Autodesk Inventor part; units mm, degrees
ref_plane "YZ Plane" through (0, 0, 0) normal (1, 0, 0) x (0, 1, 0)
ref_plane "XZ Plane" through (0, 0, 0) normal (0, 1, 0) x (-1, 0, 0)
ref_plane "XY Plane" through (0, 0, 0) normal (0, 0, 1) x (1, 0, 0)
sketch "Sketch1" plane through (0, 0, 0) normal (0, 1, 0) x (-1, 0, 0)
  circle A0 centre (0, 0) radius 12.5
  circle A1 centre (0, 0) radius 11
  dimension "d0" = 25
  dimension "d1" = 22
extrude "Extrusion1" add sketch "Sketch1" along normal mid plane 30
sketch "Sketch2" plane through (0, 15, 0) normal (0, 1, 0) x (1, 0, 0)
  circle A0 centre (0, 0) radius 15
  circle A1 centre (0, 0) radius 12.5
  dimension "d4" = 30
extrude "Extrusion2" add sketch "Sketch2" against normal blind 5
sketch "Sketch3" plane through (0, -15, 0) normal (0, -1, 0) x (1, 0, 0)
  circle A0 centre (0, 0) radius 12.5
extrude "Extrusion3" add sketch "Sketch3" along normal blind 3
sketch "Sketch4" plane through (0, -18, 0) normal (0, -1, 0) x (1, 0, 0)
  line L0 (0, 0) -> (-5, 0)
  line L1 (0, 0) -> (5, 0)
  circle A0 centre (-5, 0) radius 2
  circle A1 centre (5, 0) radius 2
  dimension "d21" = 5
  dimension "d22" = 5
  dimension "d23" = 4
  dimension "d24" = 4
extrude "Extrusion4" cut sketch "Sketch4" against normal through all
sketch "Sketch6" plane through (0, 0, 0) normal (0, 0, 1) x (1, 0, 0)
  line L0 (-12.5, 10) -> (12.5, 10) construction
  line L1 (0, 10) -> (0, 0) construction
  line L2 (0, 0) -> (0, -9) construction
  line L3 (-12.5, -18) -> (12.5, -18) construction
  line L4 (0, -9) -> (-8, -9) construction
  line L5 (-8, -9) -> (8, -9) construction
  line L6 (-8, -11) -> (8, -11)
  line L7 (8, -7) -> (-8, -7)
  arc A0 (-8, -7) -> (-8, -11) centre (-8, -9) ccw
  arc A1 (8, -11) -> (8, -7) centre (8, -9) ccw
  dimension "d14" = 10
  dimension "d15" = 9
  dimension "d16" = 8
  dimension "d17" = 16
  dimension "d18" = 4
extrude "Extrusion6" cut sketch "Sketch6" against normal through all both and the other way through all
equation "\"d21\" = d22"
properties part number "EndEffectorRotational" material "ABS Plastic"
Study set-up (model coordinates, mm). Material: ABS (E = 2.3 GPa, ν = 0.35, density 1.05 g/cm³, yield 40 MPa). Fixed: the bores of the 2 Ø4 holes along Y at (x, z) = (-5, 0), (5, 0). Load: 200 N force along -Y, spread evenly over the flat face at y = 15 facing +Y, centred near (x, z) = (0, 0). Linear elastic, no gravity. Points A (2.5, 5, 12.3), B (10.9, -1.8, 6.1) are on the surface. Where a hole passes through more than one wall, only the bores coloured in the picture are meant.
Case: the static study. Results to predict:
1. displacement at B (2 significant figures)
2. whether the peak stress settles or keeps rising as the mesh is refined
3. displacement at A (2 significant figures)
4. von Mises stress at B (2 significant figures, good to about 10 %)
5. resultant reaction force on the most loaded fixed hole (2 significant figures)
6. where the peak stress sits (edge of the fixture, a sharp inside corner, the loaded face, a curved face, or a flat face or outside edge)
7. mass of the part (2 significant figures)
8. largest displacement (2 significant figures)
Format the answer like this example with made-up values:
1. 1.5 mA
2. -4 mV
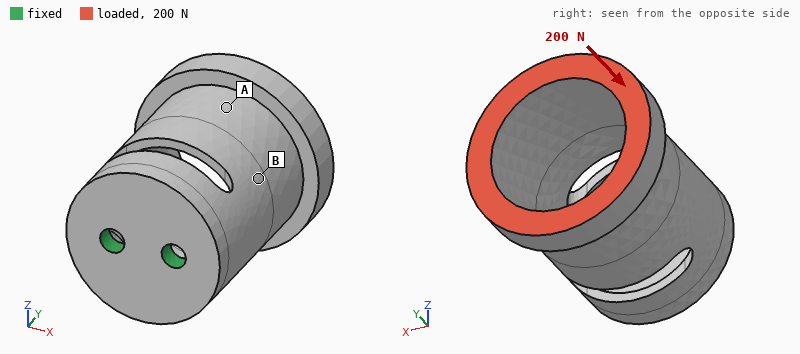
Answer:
1. 0.096 mm
2. keeps rising
3. 0.13 mm
4. 4.6 MPa
5. 100 N
6. edge of the fixture
7. 5.8 g
8. 0.16 mm
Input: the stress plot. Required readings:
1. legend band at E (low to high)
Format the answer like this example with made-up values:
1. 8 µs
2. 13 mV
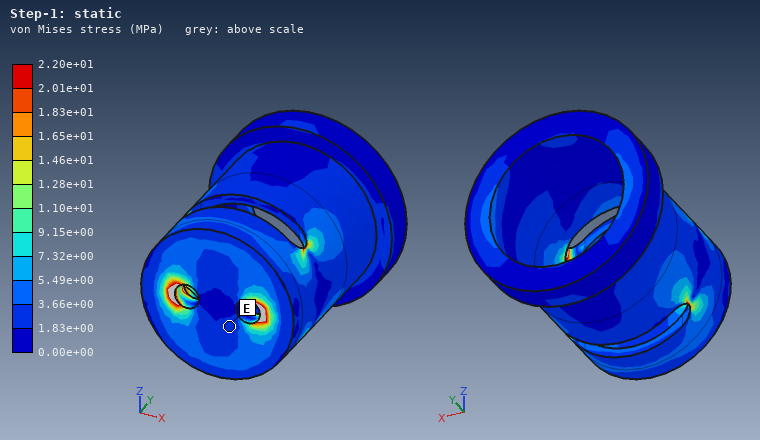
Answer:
1. 1.83e+00 to 3.66e+00 MPa
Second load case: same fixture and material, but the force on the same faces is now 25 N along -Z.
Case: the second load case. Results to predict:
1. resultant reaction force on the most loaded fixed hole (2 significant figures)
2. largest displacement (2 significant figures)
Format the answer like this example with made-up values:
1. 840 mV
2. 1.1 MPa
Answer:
1. 13 N
2. 0.46 mm
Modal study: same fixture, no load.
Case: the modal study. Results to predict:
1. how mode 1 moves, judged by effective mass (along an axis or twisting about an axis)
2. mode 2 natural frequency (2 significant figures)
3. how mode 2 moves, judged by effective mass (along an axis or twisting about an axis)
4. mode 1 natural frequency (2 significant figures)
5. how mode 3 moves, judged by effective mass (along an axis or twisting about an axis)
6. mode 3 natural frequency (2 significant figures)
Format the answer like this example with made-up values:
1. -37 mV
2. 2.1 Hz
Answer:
1. along Z
2. 1100 Hz
3. along X
4. 800 Hz
5. twisting about Y
6. 2200 Hz
